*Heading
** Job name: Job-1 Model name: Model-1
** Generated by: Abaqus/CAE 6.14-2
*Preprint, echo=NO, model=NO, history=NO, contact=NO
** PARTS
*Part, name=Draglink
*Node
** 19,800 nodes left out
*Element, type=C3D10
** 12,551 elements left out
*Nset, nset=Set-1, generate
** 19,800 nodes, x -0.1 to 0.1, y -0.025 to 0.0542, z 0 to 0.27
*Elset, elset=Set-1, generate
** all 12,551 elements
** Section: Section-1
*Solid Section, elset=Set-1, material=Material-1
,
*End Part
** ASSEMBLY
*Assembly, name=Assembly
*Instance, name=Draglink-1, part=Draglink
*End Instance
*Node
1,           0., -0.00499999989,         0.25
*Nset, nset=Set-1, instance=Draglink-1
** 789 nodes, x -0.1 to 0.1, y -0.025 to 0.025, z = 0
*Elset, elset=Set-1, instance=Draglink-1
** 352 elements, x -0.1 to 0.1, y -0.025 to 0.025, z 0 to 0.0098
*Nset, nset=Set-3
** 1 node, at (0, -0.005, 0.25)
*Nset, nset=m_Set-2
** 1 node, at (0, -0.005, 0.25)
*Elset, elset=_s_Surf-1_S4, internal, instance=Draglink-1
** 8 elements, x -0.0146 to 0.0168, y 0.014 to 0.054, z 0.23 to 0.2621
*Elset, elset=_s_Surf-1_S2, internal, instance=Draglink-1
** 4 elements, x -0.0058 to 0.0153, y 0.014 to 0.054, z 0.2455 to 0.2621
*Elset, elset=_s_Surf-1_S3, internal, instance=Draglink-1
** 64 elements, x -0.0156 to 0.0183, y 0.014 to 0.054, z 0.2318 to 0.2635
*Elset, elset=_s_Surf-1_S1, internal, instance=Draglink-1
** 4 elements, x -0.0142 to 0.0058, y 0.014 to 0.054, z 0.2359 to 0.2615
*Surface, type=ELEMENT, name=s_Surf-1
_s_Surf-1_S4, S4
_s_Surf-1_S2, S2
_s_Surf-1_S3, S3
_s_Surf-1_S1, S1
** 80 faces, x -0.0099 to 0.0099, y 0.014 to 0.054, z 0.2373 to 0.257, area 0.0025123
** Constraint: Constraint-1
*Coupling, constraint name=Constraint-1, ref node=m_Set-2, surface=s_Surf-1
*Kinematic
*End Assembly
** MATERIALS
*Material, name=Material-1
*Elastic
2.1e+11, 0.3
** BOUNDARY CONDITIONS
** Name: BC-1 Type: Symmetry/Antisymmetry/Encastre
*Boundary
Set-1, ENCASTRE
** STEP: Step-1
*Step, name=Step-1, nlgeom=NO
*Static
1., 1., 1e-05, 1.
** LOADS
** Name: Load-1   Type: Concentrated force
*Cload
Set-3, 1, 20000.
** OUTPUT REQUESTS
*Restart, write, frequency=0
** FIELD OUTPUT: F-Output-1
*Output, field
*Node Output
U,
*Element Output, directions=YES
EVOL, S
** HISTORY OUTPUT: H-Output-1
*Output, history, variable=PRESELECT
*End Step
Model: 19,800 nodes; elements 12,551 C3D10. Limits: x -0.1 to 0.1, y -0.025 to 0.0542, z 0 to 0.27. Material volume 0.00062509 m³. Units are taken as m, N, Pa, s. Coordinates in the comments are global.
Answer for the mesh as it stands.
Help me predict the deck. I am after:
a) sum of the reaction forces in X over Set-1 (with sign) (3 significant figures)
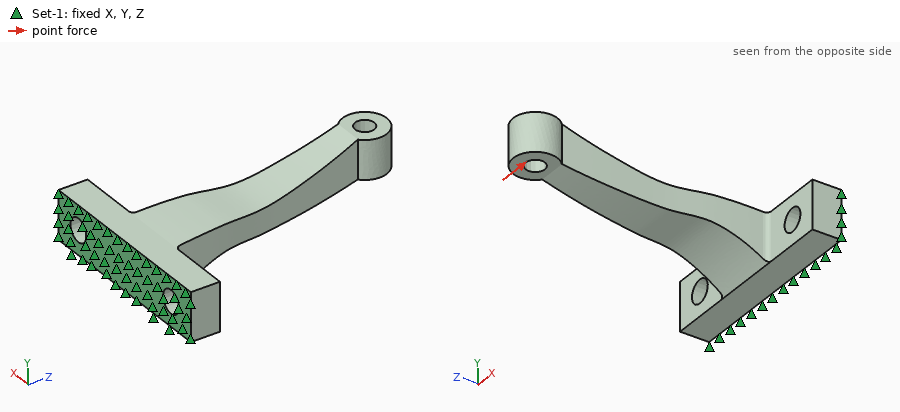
-20000 N
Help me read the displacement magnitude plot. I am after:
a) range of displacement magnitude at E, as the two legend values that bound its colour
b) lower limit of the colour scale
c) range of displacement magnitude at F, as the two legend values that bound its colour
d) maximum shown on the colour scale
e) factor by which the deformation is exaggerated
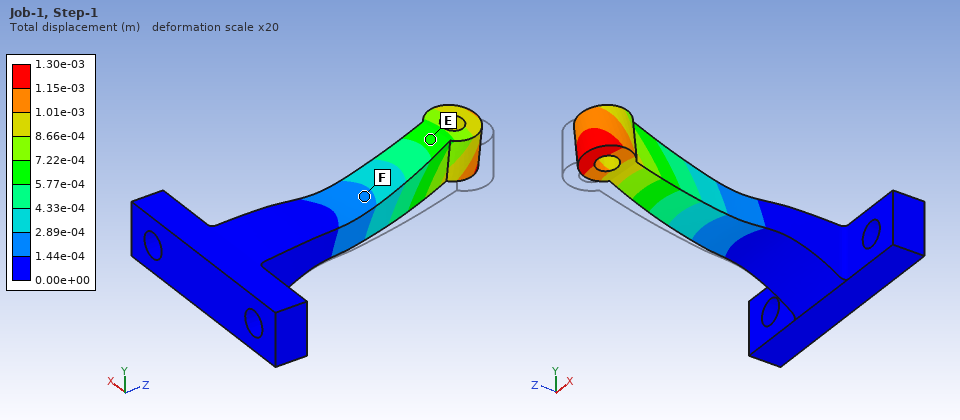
5.77e-04 to 7.22e-04 m
0.00e+00 m
1.44e-04 to 2.89e-04 m
1.30e-03 m
20
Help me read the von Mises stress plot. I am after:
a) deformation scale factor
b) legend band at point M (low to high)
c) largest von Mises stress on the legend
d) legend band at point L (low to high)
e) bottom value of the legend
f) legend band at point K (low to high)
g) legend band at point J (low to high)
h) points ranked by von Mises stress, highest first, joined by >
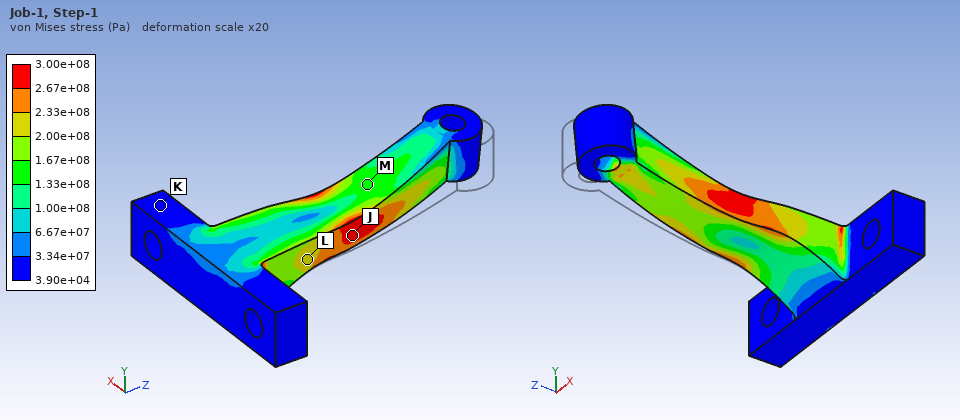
20
1.33e+08 to 1.67e+08 Pa
3.00e+08 Pa
2.00e+08 to 2.33e+08 Pa
3.90e+04 Pa
3.90e+04 to 3.34e+07 Pa
2.67e+08 to 3.00e+08 Pa
J > L > M > K
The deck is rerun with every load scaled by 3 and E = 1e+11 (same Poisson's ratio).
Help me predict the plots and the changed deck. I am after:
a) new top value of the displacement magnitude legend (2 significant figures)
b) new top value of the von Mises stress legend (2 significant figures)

0.0082 m
9.0e+08 Pa
